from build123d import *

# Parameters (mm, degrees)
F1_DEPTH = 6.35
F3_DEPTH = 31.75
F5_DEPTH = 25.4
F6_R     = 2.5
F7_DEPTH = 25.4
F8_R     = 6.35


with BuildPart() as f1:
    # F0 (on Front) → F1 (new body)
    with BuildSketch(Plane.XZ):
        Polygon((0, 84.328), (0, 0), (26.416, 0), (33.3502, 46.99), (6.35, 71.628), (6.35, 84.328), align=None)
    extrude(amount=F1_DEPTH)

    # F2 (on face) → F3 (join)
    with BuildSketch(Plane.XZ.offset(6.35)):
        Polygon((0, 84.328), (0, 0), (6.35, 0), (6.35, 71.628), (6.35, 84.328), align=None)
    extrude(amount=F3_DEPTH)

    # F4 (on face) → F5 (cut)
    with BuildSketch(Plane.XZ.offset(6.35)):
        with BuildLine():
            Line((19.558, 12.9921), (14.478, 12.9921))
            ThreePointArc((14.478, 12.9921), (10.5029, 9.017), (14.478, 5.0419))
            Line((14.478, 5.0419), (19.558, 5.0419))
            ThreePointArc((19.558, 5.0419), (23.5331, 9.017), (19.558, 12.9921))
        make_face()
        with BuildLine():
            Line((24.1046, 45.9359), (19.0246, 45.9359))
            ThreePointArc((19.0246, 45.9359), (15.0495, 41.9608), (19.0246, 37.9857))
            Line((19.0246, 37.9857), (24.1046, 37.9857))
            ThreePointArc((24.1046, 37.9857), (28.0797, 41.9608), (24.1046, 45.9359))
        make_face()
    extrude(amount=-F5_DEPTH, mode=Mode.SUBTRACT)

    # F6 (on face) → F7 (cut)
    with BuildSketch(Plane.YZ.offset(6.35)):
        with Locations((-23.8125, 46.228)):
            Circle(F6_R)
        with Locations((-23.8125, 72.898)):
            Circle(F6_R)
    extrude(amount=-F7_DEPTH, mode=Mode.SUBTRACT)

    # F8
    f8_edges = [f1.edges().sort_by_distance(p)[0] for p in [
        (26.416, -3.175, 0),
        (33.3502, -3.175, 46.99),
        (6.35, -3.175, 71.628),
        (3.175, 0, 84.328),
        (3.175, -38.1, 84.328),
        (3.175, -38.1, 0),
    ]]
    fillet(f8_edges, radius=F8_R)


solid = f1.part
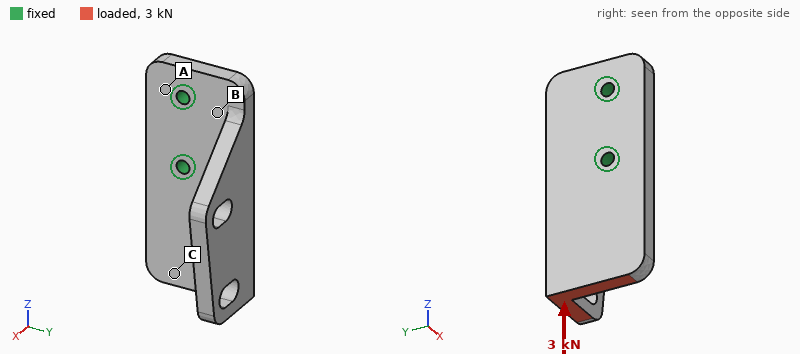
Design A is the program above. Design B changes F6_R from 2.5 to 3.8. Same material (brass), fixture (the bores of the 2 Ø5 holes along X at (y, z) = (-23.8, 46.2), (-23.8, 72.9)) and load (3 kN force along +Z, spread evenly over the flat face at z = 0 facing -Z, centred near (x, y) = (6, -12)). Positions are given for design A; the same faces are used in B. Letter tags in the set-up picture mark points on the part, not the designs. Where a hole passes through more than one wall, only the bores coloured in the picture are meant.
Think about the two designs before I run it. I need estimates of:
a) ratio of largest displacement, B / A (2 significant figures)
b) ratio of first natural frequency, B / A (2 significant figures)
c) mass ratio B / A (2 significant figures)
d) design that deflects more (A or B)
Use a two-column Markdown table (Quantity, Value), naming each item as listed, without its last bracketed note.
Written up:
| Quantity | Value |
|---|---|
| ratio of largest displacement, B / A | 0.85 |
| ratio of first natural frequency, B / A | 1.1 |
| mass ratio B / A | 0.99 |
| design that deflects more | A |
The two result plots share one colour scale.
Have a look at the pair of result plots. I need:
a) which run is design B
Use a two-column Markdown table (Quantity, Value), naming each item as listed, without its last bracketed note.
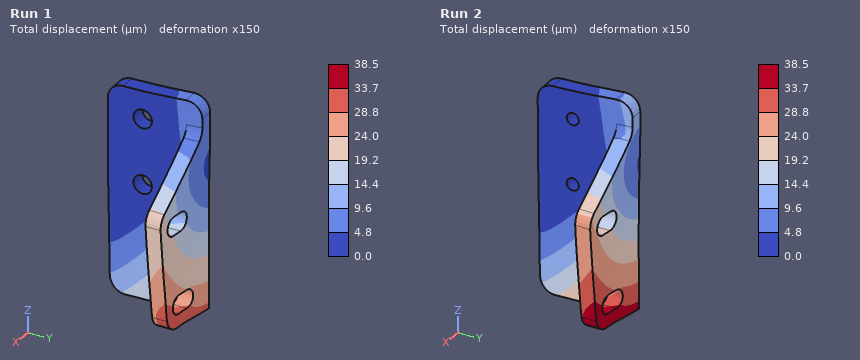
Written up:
| Quantity | Value |
|---|---|
| which run is design B | Run 1 |
